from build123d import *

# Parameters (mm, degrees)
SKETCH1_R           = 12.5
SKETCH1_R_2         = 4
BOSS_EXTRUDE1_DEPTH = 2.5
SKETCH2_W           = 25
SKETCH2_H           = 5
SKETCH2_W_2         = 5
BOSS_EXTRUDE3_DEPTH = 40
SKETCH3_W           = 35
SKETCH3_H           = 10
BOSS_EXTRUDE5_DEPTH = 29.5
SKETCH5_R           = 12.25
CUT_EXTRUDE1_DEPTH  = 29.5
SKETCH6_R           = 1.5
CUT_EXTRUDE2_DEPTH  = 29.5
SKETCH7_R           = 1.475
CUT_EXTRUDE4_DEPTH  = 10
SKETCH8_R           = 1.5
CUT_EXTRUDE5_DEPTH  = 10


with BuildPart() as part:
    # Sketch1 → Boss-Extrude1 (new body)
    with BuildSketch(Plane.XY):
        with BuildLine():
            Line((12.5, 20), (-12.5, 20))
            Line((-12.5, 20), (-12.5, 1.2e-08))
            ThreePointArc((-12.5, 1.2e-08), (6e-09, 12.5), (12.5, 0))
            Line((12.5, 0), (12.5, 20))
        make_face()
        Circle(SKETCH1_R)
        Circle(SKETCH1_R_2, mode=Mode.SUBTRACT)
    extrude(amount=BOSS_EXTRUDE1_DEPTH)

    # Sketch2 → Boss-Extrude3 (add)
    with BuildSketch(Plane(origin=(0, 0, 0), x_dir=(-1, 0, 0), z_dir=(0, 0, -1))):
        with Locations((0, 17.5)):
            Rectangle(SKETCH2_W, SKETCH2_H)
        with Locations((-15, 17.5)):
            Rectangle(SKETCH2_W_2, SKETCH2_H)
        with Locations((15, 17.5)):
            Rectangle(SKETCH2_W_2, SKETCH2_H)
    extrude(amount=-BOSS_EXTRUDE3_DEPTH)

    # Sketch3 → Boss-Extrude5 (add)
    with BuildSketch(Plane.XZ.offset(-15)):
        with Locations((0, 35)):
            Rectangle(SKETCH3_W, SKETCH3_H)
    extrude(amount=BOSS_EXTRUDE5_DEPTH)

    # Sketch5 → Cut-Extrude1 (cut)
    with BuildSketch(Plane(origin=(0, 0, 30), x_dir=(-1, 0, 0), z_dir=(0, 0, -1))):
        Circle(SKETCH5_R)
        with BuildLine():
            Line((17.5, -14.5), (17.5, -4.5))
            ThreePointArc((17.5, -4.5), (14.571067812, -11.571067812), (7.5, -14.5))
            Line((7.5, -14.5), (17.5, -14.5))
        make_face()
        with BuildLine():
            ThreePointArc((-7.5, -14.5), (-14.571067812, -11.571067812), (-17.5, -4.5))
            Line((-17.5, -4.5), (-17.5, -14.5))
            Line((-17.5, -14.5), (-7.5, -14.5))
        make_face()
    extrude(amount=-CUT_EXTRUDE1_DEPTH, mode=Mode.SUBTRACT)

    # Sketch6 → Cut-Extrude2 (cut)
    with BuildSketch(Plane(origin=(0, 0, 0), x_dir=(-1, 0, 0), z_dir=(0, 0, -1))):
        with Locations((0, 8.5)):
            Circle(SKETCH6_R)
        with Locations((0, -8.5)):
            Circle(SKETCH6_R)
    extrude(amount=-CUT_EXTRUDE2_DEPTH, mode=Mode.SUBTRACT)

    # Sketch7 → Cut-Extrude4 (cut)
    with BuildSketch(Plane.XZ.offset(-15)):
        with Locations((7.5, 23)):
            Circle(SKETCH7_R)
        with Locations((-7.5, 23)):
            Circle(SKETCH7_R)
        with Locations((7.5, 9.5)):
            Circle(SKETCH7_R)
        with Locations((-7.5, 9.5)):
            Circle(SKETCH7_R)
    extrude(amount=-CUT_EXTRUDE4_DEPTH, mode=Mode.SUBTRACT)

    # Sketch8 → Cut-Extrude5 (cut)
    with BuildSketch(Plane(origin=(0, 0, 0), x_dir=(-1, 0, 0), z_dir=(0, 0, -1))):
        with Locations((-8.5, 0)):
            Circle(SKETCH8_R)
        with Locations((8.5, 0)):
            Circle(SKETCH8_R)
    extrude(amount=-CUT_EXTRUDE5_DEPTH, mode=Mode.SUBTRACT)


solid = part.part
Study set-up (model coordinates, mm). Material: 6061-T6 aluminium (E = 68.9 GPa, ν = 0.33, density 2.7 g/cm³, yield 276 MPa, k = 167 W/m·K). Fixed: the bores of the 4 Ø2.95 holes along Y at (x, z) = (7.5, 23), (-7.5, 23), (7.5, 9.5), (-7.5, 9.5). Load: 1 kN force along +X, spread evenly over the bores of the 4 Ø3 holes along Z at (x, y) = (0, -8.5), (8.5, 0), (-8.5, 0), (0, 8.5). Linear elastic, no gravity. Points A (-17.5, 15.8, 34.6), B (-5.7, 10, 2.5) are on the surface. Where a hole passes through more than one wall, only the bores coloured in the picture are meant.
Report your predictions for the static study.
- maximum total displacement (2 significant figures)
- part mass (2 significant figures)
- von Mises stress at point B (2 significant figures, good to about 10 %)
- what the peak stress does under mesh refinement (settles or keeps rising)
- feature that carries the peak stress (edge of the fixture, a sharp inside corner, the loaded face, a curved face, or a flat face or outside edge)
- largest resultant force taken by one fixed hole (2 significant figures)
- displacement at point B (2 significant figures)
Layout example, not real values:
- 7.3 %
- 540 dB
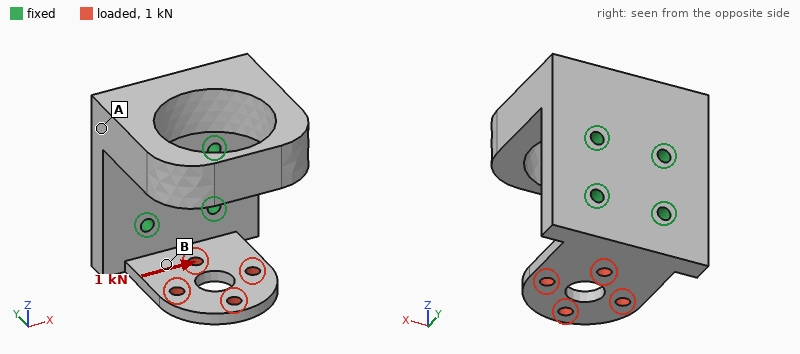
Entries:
- 96 µm
- 36 g
- 48 MPa
- keeps rising
- edge of the fixture
- 1.2 kN
- 26 µm
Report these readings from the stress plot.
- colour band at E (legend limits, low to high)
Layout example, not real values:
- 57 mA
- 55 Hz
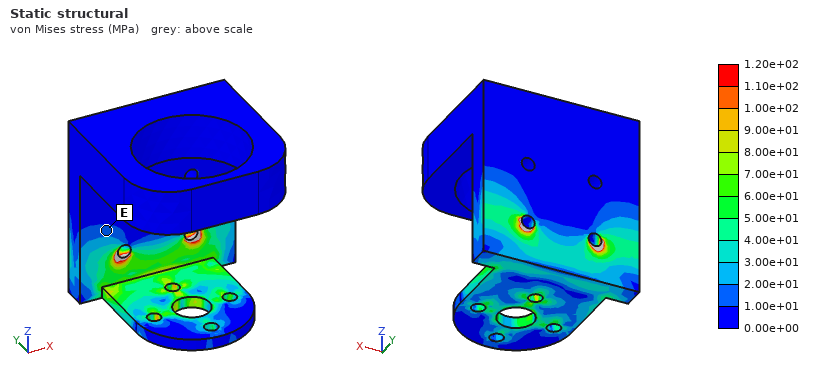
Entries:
- 1.00e+01 to 2.00e+01 MPa
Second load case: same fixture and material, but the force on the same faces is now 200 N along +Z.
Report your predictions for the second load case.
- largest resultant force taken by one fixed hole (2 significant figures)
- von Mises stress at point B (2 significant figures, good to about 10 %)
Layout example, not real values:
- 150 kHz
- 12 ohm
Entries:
- 110 N
- 76 MPa
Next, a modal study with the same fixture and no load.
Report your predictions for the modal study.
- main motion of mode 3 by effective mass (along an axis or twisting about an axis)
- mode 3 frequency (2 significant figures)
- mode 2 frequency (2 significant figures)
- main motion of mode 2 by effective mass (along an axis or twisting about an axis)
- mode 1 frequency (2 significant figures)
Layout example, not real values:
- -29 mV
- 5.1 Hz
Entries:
- along X
- 4900 Hz
- 3000 Hz
- along Z
- 2900 Hz
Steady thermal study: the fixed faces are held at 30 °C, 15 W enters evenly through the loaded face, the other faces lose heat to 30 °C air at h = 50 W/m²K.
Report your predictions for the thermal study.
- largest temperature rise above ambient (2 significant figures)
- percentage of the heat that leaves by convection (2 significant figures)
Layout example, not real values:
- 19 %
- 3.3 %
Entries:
- 33 K
- 10 %
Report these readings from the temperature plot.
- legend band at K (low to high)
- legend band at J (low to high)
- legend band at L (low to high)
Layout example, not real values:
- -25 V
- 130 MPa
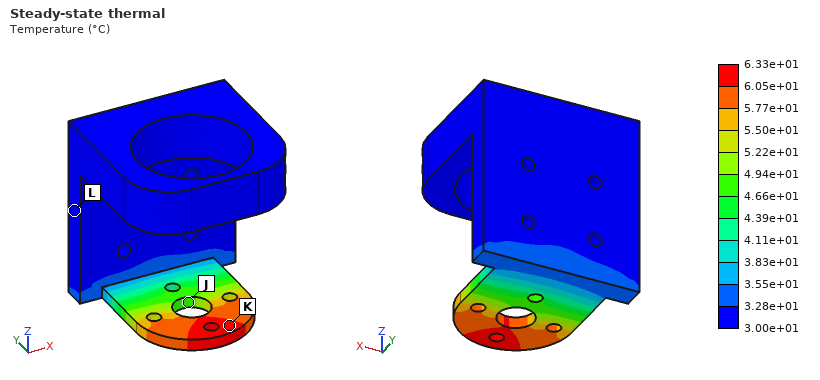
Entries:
- 6.05e+01 to 6.33e+01 °C
- 4.66e+01 to 4.94e+01 °C
- 3.00e+01 to 3.28e+01 °C
